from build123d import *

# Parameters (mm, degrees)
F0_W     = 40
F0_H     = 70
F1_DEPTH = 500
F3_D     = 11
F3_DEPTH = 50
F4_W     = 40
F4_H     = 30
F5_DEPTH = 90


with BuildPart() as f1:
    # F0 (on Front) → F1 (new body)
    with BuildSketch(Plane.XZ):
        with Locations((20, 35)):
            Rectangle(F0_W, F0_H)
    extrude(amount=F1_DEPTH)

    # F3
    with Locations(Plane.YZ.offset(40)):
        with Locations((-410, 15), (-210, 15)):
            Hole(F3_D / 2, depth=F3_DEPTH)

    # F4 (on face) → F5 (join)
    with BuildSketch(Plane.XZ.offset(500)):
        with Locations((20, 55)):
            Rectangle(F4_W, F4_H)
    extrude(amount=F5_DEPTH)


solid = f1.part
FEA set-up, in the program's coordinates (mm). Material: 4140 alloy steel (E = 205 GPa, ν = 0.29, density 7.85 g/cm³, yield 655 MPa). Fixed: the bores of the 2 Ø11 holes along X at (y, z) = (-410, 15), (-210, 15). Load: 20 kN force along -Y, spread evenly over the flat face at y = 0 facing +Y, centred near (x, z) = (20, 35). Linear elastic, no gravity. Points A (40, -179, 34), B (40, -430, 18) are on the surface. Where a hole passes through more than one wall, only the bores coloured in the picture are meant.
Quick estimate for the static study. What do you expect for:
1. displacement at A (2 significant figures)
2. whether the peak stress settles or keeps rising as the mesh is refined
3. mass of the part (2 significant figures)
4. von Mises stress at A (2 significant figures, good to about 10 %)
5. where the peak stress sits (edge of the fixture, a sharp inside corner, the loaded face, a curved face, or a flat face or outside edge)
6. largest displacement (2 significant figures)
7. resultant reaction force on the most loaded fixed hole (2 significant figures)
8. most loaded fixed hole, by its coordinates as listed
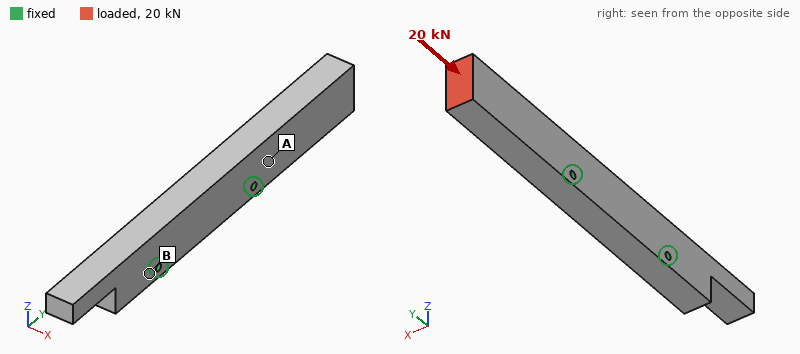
3.4 µm
keeps rising
12 kg
7.2 MPa
edge of the fixture
19 µm
16 kN
(-210, 15)
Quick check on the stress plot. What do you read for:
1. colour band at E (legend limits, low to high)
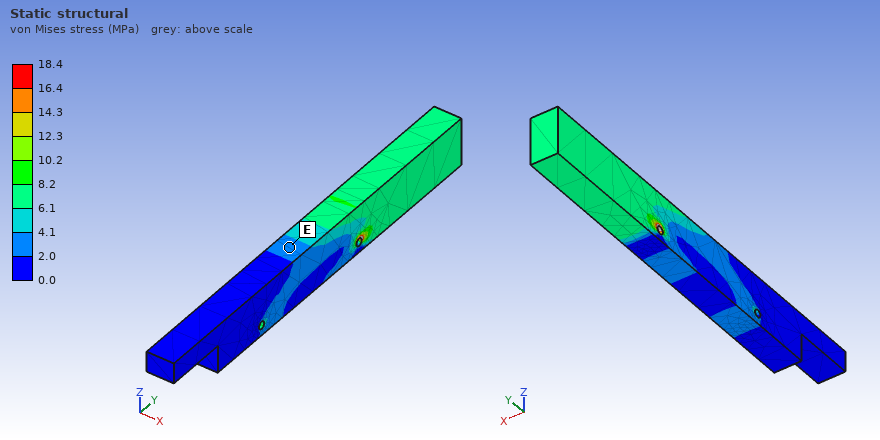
2.0 to 4.1 MPa
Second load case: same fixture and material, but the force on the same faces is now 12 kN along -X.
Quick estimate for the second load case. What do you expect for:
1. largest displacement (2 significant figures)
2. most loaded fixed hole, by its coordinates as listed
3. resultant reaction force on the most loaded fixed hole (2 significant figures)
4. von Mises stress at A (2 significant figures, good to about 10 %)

0.58 mm
(-210, 15)
16 kN
110 MPa
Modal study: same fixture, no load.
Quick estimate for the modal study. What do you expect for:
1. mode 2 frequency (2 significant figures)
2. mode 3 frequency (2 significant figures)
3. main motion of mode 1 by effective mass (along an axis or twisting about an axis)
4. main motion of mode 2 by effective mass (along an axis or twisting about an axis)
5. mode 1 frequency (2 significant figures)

940 Hz
1200 Hz
along X
along Z
660 Hz
